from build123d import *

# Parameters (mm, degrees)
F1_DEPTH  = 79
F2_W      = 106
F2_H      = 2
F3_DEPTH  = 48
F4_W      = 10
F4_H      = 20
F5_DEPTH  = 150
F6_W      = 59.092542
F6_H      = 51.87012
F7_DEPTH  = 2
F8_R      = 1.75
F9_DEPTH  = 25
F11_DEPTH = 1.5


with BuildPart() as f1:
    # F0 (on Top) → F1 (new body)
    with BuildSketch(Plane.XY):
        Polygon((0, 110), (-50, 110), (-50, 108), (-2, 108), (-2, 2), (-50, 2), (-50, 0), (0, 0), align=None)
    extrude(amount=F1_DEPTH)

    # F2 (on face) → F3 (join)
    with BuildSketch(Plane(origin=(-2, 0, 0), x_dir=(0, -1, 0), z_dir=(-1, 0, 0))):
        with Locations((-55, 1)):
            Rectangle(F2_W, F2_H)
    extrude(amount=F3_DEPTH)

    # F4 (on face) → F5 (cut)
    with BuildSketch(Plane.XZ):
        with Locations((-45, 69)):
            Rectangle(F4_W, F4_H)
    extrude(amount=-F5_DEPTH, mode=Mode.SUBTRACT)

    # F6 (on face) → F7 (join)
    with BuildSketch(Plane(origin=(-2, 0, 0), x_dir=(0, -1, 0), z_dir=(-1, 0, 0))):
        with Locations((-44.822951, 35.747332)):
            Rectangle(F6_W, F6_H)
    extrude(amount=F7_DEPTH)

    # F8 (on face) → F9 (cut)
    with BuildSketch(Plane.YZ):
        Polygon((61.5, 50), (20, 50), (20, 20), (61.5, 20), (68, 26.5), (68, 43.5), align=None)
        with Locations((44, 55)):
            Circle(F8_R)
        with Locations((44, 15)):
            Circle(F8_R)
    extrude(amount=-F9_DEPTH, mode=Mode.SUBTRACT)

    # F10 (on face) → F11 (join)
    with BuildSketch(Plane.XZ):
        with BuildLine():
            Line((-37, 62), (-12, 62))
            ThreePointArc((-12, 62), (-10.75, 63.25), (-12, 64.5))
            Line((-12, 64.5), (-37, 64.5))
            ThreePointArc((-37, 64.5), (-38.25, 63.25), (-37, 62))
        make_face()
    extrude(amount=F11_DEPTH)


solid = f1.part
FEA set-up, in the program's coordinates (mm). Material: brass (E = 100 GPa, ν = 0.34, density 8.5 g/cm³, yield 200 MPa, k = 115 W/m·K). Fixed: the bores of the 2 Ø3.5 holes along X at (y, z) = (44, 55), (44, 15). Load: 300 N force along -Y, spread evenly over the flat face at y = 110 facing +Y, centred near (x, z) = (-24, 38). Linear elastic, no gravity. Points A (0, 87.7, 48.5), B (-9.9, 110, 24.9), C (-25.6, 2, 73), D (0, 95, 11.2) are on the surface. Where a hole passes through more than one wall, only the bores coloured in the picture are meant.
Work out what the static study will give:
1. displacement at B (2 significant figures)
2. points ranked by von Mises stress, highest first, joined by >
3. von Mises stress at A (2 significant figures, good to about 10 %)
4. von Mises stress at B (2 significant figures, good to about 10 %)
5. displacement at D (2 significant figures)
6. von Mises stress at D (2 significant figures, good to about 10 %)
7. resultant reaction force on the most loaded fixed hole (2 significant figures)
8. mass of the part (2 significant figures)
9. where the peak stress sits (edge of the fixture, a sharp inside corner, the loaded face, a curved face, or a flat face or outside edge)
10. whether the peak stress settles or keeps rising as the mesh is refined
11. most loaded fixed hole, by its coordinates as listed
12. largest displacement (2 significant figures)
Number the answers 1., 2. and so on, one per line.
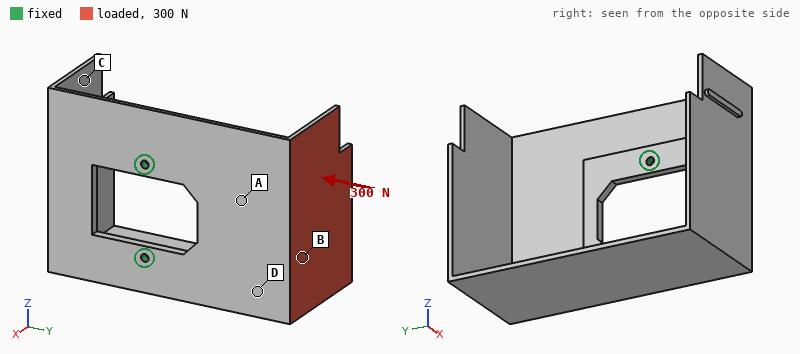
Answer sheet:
1. 0.33 mm
2. B > A > D > C
3. 28 MPa
4. 41 MPa
5. 0.21 mm
6. 15 MPa
7. 160 N
8. 360 g
9. edge of the fixture
10. keeps rising
11. (44, 55)
12. 1.0 mm
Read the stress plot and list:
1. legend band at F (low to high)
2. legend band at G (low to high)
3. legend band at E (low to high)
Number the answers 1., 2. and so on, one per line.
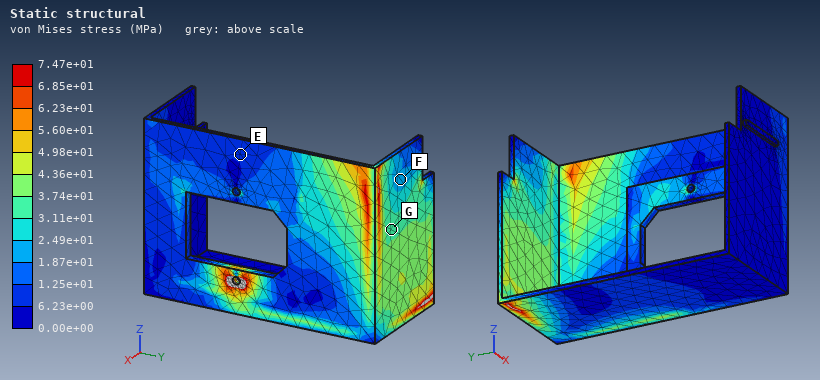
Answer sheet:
1. 1.87e+01 to 2.49e+01 MPa
2. 3.11e+01 to 3.74e+01 MPa
3. 6.23e+00 to 1.25e+01 MPa
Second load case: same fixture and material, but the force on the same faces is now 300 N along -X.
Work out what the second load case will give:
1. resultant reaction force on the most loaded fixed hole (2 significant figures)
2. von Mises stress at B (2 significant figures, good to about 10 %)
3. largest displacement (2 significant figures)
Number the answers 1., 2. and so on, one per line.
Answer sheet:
1. 170 N
2. 35 MPa
3. 1.6 mm
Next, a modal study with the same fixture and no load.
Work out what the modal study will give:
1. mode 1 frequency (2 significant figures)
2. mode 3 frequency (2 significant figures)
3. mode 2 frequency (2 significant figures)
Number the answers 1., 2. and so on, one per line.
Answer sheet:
1. 250 Hz
2. 420 Hz
3. 300 Hz
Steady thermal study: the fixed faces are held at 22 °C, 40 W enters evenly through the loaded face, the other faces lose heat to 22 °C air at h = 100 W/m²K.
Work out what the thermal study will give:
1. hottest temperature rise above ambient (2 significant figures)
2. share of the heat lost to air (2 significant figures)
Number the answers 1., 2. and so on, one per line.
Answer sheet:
1. 49 K
2. 89 %
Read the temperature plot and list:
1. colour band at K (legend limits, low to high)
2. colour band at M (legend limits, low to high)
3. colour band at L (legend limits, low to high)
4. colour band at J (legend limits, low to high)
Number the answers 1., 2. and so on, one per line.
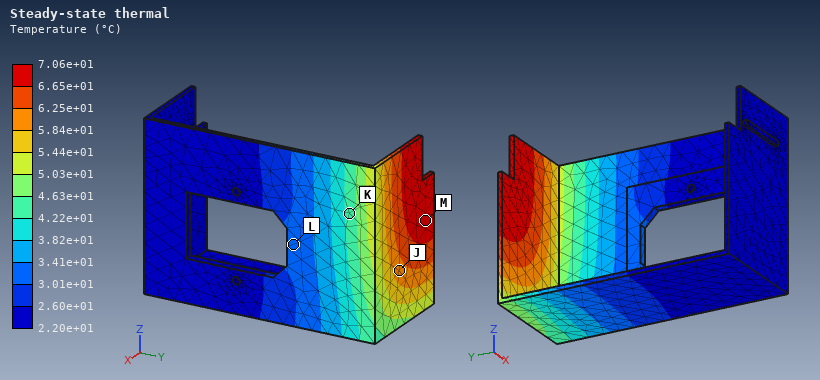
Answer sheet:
1. 4.22e+01 to 4.63e+01 °C
2. 6.65e+01 to 7.06e+01 °C
3. 3.01e+01 to 3.41e+01 °C
4. 5.84e+01 to 6.25e+01 °C
